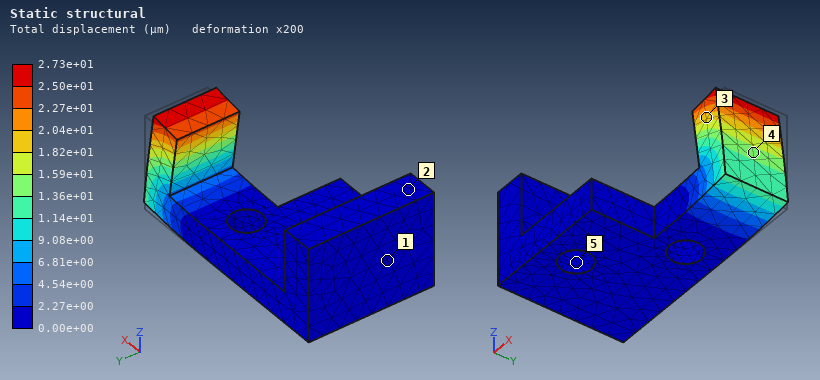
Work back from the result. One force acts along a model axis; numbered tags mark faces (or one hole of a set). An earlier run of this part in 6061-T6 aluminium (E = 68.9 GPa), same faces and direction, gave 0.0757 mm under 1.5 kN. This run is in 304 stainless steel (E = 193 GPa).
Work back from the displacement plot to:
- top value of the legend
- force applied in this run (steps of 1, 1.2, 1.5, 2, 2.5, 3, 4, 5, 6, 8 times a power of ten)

2.73e+01 µm
1.5 kN
